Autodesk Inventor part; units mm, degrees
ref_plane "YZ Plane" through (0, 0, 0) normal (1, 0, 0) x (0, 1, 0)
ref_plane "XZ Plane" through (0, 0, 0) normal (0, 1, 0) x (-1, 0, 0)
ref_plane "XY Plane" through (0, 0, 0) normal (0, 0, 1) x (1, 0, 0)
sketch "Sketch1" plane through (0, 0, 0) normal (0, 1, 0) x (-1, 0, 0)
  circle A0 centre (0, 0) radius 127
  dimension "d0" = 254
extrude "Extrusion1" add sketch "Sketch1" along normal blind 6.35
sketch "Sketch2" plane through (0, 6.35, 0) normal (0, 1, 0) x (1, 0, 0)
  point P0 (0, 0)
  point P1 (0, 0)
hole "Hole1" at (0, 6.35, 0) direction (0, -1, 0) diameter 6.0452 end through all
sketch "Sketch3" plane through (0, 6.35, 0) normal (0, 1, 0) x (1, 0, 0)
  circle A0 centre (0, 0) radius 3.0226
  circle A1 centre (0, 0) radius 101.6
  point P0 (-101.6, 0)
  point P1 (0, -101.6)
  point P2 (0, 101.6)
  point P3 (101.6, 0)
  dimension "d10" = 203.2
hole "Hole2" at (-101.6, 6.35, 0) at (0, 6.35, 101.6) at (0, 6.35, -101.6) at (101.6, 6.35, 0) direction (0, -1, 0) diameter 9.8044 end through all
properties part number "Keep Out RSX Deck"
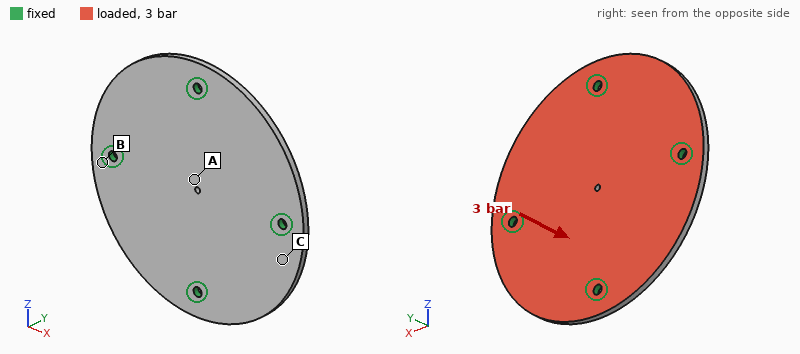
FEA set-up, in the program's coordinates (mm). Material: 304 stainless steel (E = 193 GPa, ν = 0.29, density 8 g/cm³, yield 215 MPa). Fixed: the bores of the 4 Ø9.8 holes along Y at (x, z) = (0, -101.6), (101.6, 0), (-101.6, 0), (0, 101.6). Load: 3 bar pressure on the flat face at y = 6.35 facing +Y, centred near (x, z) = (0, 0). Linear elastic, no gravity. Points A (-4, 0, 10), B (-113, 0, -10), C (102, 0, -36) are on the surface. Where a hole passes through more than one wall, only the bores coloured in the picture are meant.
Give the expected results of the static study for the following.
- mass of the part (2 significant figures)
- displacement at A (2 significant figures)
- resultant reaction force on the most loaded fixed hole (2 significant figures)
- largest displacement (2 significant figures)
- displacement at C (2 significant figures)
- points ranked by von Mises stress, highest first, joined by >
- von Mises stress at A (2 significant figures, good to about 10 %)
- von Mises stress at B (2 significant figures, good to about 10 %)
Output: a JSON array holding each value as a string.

["2.6 kg", "0.17 mm", "3.8 kN", "0.17 mm", "0.052 mm", "B > A > C", "35 MPa", "53 MPa"]
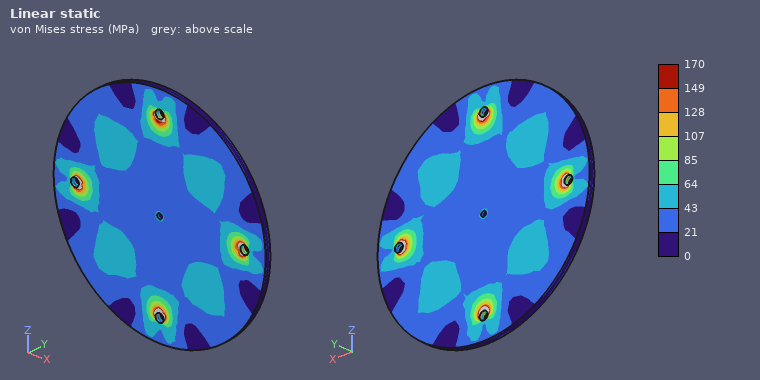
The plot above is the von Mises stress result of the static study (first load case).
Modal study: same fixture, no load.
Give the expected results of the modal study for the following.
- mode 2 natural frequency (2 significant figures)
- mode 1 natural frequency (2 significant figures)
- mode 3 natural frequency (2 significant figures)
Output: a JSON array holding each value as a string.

["1100 Hz", "1100 Hz", "1200 Hz"]
